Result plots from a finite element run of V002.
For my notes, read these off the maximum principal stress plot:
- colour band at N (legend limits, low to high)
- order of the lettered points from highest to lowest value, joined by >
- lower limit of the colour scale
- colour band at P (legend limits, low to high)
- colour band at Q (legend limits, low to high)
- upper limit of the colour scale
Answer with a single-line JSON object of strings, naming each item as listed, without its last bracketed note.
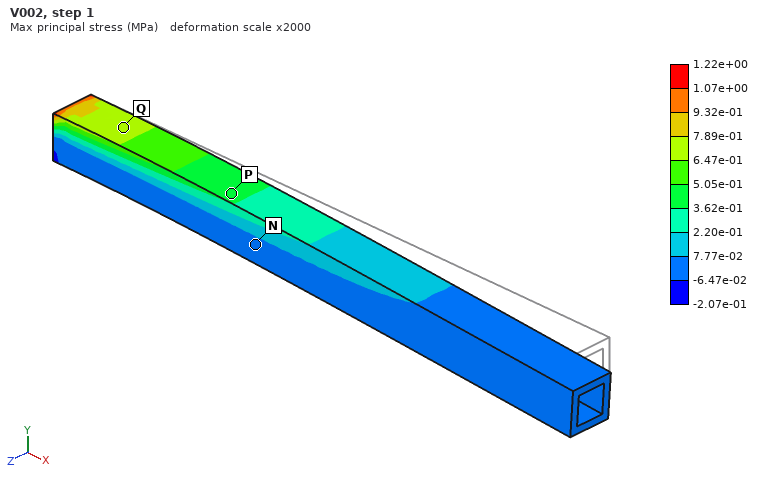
{"colour band at N": "-6.47e-02 to 7.77e-02 MPa", "order of the lettered points from highest to lowest value, joined by >": "Q > P > N", "lower limit of the colour scale": "-2.07e-01 MPa", "colour band at P": "3.62e-01 to 5.05e-01 MPa", "colour band at Q": "6.47e-01 to 7.89e-01 MPa", "upper limit of the colour scale": "1.22e+00 MPa"}
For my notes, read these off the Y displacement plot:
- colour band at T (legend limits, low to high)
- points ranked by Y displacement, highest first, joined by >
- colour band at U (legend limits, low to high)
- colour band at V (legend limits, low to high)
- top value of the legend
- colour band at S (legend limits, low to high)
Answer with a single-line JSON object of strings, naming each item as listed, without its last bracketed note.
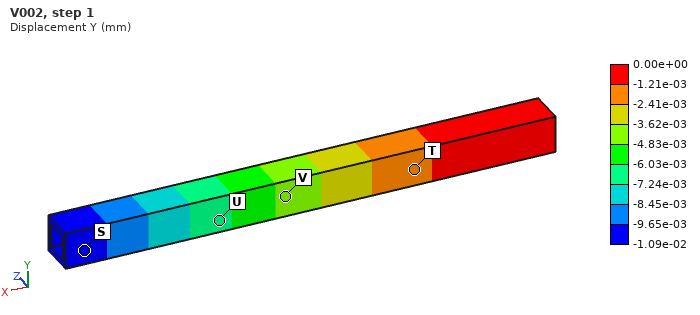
{"colour band at T": "-2.41e-03 to -1.21e-03 mm", "points ranked by Y displacement, highest first, joined by >": "T > V > U > S", "colour band at U": "-7.24e-03 to -6.03e-03 mm", "colour band at V": "-4.83e-03 to -3.62e-03 mm", "top value of the legend": "0.00e+00 mm", "colour band at S": "-1.09e-02 to -9.65e-03 mm"}
